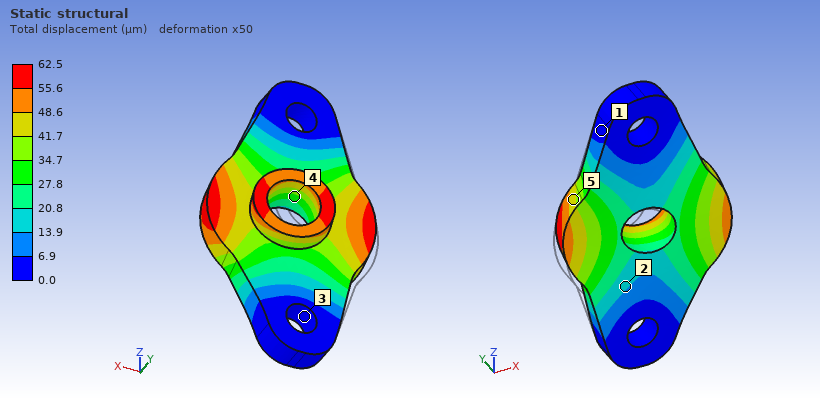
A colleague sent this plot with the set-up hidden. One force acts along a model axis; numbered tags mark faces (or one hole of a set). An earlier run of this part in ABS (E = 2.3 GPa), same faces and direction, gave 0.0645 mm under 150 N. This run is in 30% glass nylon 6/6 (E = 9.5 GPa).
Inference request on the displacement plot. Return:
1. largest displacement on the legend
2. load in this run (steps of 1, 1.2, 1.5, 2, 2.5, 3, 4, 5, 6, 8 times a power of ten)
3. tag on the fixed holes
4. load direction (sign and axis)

62.5 µm
600 N
3
+X
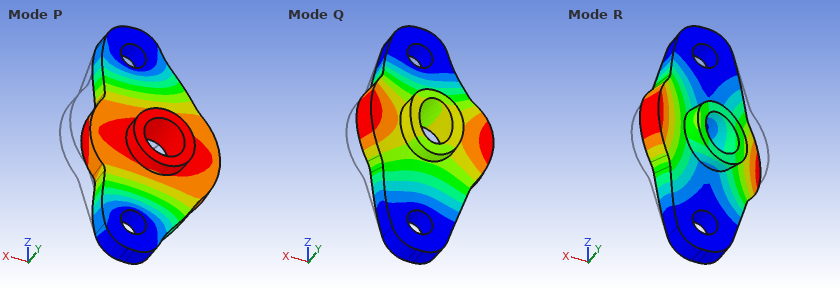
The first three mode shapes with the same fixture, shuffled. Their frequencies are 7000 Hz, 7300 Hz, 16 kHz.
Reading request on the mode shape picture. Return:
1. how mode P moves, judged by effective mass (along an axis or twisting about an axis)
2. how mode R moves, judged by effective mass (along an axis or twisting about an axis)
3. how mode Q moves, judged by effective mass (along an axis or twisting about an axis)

along X
twisting about Z
along Y
